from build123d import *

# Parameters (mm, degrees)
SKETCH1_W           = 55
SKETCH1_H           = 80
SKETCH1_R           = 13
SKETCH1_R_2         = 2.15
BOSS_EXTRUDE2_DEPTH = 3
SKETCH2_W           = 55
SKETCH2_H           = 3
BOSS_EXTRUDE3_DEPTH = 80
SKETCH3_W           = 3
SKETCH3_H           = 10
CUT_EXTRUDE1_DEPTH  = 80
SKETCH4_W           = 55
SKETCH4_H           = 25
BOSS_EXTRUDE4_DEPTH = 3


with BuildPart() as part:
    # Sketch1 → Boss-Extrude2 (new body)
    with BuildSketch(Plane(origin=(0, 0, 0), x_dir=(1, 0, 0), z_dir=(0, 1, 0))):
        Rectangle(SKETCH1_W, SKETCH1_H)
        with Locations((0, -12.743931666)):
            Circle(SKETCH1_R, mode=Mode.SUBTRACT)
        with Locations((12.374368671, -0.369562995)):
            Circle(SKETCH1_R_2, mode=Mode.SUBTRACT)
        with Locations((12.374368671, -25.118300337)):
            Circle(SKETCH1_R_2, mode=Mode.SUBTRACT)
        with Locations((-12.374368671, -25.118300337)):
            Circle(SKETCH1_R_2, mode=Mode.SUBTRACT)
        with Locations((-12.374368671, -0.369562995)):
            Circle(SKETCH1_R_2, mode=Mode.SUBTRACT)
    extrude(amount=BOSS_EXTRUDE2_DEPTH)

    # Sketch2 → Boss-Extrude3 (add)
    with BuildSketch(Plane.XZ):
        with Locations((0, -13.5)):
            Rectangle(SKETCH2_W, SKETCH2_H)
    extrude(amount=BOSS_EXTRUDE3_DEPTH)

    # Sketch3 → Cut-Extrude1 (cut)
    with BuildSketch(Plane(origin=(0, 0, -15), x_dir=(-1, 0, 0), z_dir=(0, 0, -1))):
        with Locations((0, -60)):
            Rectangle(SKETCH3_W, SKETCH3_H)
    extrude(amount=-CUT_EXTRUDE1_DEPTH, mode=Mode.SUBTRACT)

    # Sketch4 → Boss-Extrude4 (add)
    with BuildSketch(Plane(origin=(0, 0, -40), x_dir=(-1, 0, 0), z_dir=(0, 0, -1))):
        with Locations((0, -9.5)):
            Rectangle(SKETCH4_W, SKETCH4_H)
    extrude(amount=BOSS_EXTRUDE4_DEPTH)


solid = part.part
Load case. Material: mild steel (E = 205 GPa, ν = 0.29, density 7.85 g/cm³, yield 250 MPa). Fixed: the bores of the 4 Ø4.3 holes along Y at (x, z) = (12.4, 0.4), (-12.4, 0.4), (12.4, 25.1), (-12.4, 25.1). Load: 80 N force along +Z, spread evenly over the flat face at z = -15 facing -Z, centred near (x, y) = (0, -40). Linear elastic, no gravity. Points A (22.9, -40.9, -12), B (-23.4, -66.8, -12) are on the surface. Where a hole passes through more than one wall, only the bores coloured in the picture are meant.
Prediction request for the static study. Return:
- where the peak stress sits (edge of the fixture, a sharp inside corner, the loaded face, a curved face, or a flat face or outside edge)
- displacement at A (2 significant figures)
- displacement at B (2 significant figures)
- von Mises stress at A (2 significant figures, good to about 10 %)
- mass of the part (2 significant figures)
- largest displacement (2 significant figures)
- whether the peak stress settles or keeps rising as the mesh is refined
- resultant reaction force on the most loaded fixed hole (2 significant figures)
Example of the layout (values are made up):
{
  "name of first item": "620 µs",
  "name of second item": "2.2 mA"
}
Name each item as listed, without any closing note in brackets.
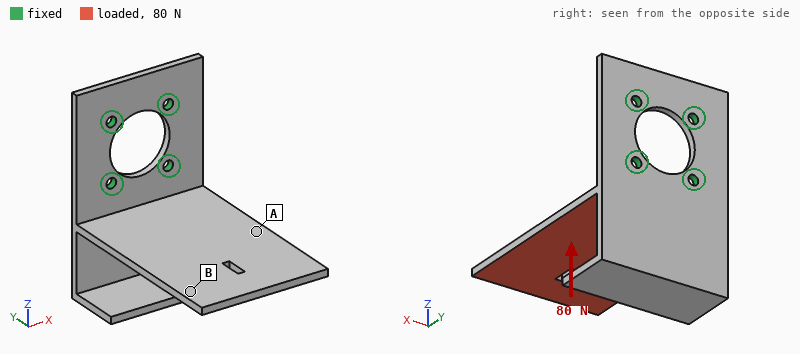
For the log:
{
  "where the peak stress sits": "edge of the fixture",
  "displacement at A": "0.15 mm",
  "displacement at B": "0.28 mm",
  "von Mises stress at A": "9.4 MPa",
  "mass of the part": "230 g",
  "largest displacement": "0.35 mm",
  "whether the peak stress settles or keeps rising as the mesh is refined": "keeps rising",
  "resultant reaction force on the most loaded fixed hole": "41 N"
}
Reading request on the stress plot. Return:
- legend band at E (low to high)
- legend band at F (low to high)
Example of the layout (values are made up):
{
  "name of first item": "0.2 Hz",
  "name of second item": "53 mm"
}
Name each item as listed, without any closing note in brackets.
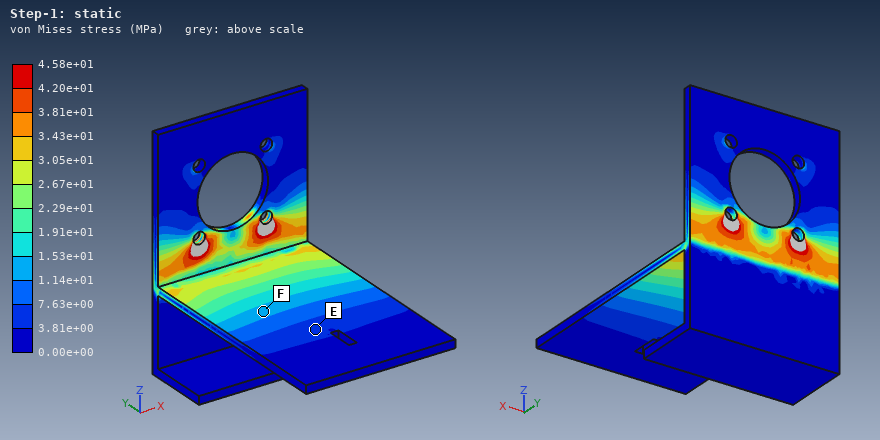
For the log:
{
  "legend band at E": "3.81e+00 to 7.63e+00 MPa",
  "legend band at F": "1.14e+01 to 1.53e+01 MPa"
}
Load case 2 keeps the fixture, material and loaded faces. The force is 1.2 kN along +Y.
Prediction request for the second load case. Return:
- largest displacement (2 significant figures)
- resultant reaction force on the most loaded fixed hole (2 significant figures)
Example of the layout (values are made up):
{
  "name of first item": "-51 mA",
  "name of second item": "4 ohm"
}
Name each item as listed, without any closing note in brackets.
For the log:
{
  "largest displacement": "0.64 mm",
  "resultant reaction force on the most loaded fixed hole": "660 N"
}
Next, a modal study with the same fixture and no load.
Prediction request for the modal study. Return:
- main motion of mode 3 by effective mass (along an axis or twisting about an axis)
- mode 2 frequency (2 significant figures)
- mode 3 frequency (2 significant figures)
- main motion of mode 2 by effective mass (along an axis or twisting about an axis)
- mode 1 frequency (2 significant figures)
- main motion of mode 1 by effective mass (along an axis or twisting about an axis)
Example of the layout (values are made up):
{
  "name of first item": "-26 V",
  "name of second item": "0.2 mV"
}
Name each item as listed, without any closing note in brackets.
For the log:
{
  "main motion of mode 3 by effective mass": "along X",
  "mode 2 frequency": "860 Hz",
  "mode 3 frequency": "930 Hz",
  "main motion of mode 2 by effective mass": "along Y",
  "mode 1 frequency": "290 Hz",
  "main motion of mode 1 by effective mass": "along Z"
}
